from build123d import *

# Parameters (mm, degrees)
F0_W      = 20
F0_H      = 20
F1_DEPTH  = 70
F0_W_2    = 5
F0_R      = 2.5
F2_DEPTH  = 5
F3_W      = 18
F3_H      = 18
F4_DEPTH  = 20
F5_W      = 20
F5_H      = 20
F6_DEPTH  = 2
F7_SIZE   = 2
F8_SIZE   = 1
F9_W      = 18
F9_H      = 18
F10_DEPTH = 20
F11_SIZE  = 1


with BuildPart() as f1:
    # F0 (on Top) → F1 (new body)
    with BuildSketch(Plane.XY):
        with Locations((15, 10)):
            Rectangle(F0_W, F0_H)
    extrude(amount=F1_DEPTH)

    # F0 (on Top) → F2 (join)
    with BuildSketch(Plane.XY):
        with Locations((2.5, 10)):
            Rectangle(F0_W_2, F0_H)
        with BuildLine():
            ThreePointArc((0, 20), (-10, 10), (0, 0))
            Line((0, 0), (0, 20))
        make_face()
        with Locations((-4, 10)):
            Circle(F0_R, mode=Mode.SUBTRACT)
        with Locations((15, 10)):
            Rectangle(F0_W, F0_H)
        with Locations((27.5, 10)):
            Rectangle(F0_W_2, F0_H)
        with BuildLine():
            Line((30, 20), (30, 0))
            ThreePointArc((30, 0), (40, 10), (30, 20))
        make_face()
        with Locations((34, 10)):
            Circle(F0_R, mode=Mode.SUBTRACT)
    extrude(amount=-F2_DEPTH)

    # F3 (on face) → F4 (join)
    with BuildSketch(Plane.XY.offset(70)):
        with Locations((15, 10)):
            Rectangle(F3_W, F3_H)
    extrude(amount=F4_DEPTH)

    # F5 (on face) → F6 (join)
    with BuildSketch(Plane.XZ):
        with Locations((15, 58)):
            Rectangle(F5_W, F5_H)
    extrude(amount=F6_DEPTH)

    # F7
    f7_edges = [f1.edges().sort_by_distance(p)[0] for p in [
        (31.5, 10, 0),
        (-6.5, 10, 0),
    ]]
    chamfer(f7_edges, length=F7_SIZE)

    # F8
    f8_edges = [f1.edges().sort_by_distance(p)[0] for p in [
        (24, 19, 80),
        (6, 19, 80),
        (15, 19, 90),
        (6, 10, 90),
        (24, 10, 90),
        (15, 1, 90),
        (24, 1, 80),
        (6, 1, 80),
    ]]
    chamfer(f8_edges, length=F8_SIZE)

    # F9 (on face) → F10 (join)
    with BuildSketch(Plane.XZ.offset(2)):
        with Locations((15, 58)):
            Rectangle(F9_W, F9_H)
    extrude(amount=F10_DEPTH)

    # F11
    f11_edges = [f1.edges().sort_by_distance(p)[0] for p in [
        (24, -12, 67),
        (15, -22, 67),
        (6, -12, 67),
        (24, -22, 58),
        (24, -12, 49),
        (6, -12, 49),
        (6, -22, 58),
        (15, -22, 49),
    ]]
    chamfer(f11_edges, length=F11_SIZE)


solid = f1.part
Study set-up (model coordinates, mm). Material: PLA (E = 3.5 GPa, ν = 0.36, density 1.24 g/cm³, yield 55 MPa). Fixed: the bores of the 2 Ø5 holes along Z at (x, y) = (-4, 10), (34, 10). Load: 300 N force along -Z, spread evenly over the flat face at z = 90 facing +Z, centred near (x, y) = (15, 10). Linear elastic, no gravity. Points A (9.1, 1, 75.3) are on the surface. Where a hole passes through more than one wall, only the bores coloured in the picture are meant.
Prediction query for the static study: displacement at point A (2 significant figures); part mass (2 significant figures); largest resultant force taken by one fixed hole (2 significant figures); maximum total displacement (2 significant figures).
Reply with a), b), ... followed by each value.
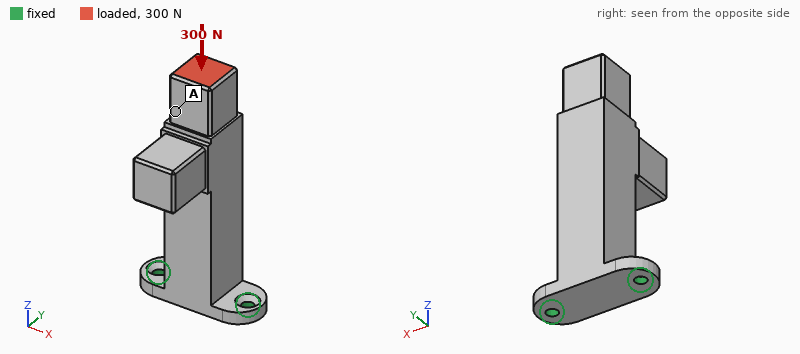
a) 64 µm
b) 57 g
c) 190 N
d) 70 µm
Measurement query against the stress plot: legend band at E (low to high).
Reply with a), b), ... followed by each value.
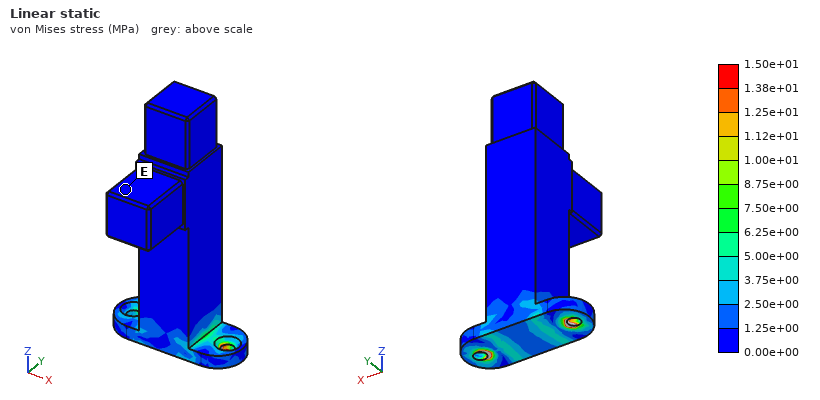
a) 0.00e+00 to 1.25e+00 MPa
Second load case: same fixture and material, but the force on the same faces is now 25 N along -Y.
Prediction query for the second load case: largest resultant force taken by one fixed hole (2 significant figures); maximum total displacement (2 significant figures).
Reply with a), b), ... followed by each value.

a) 13 N
b) 1.4 mm
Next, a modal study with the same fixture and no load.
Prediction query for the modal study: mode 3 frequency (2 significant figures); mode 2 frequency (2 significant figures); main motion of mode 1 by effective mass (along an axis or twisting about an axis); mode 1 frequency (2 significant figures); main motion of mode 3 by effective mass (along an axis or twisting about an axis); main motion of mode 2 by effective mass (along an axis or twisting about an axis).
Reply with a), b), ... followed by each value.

a) 1500 Hz
b) 380 Hz
c) along Y
d) 160 Hz
e) twisting about Z
f) along X
